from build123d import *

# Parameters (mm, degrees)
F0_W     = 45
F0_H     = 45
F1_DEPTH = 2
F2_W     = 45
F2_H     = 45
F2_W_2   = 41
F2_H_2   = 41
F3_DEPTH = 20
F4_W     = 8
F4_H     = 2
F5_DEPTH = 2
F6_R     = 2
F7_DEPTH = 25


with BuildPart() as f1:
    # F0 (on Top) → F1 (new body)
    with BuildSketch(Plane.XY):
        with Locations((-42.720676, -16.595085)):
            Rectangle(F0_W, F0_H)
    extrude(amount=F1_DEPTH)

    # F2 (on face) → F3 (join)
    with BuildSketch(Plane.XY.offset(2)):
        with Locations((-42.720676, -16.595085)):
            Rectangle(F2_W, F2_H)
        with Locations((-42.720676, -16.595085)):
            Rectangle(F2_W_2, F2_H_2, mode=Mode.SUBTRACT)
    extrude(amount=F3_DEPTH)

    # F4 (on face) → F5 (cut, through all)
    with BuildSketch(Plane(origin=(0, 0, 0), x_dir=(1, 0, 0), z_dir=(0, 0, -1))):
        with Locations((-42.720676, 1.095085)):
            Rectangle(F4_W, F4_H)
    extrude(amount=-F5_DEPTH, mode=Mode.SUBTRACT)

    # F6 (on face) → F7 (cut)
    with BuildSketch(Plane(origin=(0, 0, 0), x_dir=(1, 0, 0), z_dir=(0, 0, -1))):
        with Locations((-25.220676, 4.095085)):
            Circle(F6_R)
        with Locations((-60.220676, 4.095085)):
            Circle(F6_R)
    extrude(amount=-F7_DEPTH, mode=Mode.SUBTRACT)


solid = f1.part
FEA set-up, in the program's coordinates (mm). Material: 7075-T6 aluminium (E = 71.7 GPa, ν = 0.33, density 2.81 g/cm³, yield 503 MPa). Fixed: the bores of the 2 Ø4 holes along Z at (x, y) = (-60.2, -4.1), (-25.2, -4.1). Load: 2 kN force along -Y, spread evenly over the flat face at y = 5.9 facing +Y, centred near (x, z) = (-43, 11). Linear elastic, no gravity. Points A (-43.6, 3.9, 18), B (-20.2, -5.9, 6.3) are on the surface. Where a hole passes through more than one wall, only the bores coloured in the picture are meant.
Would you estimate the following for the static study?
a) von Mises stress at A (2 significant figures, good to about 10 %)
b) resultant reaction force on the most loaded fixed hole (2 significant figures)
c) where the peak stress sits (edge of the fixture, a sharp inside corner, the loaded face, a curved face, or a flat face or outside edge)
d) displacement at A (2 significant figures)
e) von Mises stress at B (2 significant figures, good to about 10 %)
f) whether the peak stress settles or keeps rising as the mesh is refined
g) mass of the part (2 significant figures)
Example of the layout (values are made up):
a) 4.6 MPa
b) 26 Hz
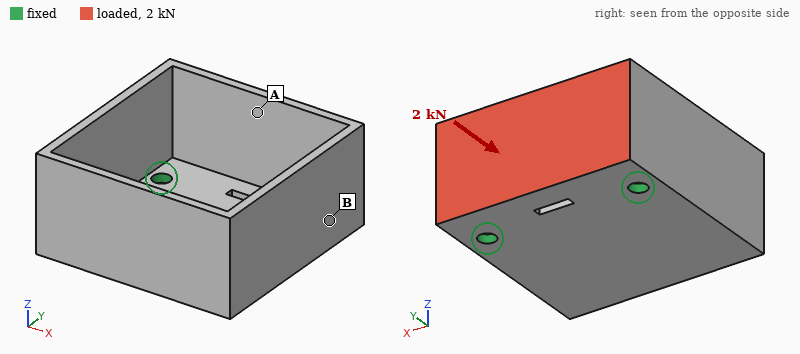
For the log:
a) 150 MPa
b) 1.0 kN
c) edge of the fixture
d) 0.60 mm
e) 69 MPa
f) keeps rising
g) 30 g
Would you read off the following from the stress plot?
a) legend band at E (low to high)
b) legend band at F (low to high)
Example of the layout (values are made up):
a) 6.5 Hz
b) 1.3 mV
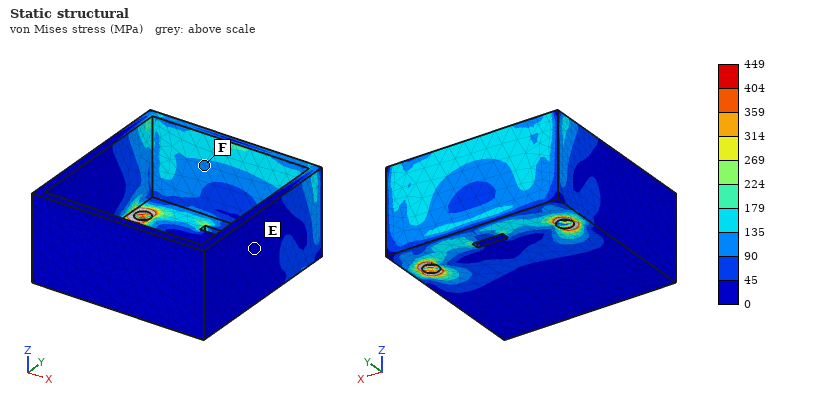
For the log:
a) 0 to 45 MPa
b) 90 to 135 MPa
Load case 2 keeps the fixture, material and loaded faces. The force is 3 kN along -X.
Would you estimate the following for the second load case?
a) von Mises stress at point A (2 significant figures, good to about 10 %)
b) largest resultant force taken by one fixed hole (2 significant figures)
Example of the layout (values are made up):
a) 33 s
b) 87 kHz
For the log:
a) 38 MPa
b) 1.8 kN
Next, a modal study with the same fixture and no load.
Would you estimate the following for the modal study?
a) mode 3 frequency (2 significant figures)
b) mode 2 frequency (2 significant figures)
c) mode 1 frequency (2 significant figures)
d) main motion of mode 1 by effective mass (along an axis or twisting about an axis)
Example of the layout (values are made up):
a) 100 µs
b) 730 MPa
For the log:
a) 5300 Hz
b) 2200 Hz
c) 1500 Hz
d) along Z
